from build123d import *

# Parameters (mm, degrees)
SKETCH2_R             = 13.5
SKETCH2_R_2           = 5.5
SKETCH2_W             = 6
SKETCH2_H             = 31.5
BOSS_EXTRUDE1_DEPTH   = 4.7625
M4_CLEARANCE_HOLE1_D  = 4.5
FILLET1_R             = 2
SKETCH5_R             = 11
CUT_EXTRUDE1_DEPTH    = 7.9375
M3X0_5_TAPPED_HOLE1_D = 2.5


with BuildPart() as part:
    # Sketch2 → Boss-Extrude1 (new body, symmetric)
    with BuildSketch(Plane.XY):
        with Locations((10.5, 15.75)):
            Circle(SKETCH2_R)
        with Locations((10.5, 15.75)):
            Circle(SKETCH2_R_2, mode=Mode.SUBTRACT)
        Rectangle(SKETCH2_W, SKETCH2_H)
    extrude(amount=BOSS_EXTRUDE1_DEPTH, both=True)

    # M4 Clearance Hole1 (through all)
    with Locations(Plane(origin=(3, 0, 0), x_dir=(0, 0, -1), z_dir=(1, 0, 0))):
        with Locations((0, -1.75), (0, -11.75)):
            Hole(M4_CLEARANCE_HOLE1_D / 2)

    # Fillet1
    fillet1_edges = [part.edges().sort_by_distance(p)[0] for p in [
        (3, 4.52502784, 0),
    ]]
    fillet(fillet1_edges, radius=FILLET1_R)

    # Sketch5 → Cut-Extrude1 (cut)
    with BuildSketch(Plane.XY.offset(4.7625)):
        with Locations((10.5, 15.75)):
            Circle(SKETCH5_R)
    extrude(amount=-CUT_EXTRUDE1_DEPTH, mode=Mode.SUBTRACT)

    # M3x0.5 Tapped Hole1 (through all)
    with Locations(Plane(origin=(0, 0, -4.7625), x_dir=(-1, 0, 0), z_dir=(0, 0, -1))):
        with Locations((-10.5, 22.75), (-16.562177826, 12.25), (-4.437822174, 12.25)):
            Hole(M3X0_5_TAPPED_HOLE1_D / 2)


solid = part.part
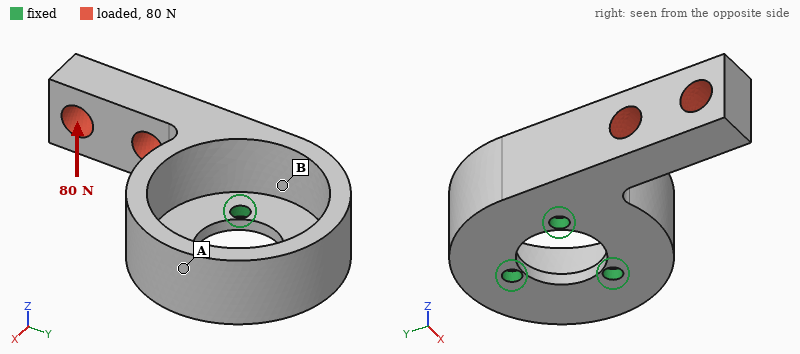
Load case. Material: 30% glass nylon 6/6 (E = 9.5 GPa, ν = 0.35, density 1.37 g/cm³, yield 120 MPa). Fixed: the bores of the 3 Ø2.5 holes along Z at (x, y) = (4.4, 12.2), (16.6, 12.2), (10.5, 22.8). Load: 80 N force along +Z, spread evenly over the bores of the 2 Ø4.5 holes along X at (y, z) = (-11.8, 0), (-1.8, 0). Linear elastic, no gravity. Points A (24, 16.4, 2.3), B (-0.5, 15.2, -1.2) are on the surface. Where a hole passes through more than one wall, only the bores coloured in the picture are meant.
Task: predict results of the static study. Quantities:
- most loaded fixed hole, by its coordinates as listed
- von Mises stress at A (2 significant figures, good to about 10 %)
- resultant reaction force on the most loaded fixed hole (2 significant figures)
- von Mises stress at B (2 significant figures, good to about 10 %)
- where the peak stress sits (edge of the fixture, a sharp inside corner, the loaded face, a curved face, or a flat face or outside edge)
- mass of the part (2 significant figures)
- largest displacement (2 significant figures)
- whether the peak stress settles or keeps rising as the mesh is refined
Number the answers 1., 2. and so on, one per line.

1. (4.4, 12.2)
2. 8.6 MPa
3. 150 N
4. 20 MPa
5. edge of the fixture
6. 4.7 g
7. 0.43 mm
8. keeps rising
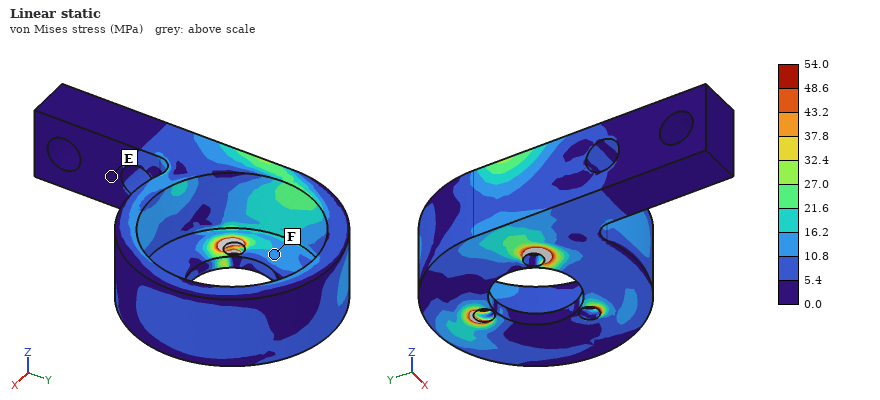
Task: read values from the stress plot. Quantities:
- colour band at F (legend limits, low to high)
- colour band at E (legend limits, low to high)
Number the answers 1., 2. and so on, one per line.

1. 10.8 to 16.2 MPa
2. 0.0 to 5.4 MPa
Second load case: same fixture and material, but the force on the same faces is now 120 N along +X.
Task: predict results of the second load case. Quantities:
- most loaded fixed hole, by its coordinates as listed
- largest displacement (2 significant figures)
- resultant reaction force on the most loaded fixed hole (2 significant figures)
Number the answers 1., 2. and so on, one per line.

1. (16.6, 12.2)
2. 0.28 mm
3. 170 N
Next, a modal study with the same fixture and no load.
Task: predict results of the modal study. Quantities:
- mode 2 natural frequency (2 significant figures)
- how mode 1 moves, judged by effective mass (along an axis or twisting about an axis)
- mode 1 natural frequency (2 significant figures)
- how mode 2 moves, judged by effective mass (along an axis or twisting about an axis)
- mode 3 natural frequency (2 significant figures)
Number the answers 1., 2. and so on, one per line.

1. 3900 Hz
2. along Z
3. 2200 Hz
4. along X
5. 5600 Hz
